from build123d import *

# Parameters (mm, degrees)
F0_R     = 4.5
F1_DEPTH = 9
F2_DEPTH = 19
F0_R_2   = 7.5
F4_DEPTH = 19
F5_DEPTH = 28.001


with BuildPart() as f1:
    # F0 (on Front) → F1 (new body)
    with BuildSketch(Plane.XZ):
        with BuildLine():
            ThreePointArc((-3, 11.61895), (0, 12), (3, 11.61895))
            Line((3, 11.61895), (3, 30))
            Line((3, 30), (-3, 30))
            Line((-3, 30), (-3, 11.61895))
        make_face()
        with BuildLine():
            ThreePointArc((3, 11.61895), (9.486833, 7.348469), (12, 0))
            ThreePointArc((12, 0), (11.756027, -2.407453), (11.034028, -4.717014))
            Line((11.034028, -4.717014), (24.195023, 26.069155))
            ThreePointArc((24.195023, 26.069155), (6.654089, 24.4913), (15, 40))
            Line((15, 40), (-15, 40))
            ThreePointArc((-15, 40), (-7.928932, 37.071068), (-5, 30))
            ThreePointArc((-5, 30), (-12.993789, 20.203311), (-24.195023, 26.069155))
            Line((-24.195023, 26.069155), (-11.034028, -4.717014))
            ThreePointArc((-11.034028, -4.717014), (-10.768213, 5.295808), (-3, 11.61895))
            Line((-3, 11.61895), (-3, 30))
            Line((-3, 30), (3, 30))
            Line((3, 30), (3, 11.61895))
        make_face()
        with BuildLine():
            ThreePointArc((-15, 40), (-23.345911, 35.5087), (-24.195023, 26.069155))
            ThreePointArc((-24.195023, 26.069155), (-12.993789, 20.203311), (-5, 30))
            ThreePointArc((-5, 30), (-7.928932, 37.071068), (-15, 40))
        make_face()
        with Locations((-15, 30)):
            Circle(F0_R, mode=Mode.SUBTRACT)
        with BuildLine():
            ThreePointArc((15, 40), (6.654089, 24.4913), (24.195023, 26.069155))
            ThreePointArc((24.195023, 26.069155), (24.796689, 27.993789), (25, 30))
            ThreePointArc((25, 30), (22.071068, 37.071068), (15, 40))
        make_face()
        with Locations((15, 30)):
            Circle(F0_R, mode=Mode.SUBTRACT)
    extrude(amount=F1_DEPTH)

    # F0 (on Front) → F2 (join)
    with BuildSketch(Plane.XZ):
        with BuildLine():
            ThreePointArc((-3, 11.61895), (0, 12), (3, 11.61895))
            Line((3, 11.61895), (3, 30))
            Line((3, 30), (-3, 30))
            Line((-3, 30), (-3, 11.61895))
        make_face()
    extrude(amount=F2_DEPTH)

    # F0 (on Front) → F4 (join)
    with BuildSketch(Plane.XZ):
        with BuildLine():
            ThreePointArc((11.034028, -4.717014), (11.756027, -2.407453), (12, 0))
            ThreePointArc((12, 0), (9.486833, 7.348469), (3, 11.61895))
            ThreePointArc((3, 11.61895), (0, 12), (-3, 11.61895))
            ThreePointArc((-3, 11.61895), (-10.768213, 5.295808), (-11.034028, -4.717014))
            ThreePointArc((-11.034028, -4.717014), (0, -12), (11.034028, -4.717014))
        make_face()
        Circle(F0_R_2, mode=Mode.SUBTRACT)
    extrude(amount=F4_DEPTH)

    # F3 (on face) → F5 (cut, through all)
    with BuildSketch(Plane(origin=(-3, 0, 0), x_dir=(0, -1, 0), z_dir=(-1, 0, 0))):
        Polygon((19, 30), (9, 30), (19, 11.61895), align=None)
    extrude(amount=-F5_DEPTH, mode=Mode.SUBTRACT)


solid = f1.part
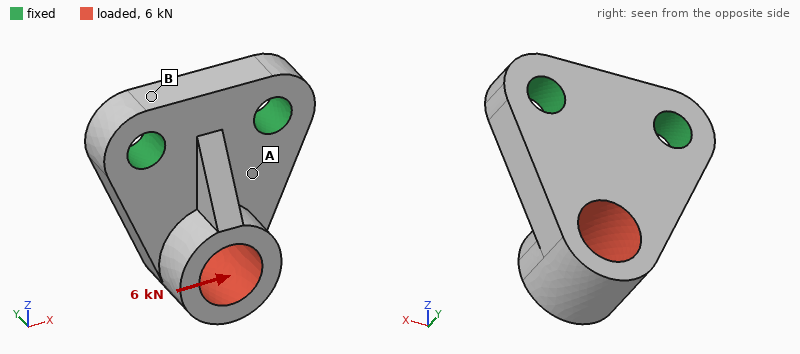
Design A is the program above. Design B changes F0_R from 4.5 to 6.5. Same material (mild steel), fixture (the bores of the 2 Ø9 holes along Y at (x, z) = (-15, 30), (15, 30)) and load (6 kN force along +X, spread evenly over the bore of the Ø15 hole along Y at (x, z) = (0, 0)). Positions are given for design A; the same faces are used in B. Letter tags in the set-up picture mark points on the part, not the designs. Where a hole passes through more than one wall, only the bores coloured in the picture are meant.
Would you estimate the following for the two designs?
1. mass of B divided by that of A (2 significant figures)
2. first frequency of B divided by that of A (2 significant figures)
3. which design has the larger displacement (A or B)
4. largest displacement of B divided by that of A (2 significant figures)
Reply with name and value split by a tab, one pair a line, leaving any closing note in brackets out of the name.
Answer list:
mass of B divided by that of A	0.93
first frequency of B divided by that of A	1.1
which design has the larger displacement	A
largest displacement of B divided by that of A	0.91
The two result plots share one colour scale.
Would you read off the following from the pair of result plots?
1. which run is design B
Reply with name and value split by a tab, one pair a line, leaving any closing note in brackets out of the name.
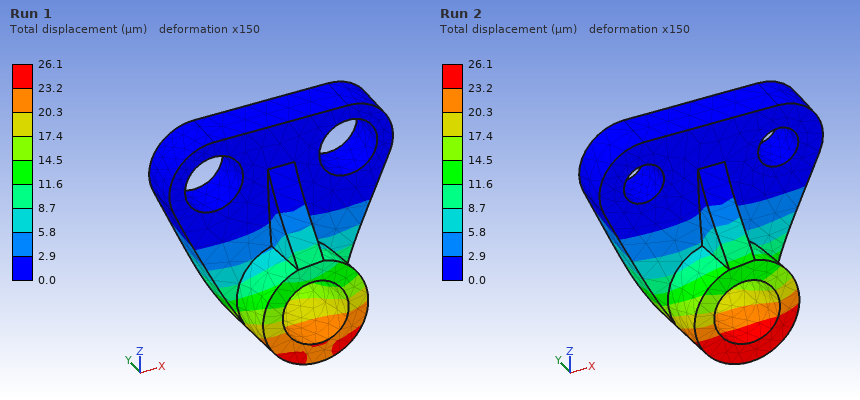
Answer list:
which run is design B	Run 1
